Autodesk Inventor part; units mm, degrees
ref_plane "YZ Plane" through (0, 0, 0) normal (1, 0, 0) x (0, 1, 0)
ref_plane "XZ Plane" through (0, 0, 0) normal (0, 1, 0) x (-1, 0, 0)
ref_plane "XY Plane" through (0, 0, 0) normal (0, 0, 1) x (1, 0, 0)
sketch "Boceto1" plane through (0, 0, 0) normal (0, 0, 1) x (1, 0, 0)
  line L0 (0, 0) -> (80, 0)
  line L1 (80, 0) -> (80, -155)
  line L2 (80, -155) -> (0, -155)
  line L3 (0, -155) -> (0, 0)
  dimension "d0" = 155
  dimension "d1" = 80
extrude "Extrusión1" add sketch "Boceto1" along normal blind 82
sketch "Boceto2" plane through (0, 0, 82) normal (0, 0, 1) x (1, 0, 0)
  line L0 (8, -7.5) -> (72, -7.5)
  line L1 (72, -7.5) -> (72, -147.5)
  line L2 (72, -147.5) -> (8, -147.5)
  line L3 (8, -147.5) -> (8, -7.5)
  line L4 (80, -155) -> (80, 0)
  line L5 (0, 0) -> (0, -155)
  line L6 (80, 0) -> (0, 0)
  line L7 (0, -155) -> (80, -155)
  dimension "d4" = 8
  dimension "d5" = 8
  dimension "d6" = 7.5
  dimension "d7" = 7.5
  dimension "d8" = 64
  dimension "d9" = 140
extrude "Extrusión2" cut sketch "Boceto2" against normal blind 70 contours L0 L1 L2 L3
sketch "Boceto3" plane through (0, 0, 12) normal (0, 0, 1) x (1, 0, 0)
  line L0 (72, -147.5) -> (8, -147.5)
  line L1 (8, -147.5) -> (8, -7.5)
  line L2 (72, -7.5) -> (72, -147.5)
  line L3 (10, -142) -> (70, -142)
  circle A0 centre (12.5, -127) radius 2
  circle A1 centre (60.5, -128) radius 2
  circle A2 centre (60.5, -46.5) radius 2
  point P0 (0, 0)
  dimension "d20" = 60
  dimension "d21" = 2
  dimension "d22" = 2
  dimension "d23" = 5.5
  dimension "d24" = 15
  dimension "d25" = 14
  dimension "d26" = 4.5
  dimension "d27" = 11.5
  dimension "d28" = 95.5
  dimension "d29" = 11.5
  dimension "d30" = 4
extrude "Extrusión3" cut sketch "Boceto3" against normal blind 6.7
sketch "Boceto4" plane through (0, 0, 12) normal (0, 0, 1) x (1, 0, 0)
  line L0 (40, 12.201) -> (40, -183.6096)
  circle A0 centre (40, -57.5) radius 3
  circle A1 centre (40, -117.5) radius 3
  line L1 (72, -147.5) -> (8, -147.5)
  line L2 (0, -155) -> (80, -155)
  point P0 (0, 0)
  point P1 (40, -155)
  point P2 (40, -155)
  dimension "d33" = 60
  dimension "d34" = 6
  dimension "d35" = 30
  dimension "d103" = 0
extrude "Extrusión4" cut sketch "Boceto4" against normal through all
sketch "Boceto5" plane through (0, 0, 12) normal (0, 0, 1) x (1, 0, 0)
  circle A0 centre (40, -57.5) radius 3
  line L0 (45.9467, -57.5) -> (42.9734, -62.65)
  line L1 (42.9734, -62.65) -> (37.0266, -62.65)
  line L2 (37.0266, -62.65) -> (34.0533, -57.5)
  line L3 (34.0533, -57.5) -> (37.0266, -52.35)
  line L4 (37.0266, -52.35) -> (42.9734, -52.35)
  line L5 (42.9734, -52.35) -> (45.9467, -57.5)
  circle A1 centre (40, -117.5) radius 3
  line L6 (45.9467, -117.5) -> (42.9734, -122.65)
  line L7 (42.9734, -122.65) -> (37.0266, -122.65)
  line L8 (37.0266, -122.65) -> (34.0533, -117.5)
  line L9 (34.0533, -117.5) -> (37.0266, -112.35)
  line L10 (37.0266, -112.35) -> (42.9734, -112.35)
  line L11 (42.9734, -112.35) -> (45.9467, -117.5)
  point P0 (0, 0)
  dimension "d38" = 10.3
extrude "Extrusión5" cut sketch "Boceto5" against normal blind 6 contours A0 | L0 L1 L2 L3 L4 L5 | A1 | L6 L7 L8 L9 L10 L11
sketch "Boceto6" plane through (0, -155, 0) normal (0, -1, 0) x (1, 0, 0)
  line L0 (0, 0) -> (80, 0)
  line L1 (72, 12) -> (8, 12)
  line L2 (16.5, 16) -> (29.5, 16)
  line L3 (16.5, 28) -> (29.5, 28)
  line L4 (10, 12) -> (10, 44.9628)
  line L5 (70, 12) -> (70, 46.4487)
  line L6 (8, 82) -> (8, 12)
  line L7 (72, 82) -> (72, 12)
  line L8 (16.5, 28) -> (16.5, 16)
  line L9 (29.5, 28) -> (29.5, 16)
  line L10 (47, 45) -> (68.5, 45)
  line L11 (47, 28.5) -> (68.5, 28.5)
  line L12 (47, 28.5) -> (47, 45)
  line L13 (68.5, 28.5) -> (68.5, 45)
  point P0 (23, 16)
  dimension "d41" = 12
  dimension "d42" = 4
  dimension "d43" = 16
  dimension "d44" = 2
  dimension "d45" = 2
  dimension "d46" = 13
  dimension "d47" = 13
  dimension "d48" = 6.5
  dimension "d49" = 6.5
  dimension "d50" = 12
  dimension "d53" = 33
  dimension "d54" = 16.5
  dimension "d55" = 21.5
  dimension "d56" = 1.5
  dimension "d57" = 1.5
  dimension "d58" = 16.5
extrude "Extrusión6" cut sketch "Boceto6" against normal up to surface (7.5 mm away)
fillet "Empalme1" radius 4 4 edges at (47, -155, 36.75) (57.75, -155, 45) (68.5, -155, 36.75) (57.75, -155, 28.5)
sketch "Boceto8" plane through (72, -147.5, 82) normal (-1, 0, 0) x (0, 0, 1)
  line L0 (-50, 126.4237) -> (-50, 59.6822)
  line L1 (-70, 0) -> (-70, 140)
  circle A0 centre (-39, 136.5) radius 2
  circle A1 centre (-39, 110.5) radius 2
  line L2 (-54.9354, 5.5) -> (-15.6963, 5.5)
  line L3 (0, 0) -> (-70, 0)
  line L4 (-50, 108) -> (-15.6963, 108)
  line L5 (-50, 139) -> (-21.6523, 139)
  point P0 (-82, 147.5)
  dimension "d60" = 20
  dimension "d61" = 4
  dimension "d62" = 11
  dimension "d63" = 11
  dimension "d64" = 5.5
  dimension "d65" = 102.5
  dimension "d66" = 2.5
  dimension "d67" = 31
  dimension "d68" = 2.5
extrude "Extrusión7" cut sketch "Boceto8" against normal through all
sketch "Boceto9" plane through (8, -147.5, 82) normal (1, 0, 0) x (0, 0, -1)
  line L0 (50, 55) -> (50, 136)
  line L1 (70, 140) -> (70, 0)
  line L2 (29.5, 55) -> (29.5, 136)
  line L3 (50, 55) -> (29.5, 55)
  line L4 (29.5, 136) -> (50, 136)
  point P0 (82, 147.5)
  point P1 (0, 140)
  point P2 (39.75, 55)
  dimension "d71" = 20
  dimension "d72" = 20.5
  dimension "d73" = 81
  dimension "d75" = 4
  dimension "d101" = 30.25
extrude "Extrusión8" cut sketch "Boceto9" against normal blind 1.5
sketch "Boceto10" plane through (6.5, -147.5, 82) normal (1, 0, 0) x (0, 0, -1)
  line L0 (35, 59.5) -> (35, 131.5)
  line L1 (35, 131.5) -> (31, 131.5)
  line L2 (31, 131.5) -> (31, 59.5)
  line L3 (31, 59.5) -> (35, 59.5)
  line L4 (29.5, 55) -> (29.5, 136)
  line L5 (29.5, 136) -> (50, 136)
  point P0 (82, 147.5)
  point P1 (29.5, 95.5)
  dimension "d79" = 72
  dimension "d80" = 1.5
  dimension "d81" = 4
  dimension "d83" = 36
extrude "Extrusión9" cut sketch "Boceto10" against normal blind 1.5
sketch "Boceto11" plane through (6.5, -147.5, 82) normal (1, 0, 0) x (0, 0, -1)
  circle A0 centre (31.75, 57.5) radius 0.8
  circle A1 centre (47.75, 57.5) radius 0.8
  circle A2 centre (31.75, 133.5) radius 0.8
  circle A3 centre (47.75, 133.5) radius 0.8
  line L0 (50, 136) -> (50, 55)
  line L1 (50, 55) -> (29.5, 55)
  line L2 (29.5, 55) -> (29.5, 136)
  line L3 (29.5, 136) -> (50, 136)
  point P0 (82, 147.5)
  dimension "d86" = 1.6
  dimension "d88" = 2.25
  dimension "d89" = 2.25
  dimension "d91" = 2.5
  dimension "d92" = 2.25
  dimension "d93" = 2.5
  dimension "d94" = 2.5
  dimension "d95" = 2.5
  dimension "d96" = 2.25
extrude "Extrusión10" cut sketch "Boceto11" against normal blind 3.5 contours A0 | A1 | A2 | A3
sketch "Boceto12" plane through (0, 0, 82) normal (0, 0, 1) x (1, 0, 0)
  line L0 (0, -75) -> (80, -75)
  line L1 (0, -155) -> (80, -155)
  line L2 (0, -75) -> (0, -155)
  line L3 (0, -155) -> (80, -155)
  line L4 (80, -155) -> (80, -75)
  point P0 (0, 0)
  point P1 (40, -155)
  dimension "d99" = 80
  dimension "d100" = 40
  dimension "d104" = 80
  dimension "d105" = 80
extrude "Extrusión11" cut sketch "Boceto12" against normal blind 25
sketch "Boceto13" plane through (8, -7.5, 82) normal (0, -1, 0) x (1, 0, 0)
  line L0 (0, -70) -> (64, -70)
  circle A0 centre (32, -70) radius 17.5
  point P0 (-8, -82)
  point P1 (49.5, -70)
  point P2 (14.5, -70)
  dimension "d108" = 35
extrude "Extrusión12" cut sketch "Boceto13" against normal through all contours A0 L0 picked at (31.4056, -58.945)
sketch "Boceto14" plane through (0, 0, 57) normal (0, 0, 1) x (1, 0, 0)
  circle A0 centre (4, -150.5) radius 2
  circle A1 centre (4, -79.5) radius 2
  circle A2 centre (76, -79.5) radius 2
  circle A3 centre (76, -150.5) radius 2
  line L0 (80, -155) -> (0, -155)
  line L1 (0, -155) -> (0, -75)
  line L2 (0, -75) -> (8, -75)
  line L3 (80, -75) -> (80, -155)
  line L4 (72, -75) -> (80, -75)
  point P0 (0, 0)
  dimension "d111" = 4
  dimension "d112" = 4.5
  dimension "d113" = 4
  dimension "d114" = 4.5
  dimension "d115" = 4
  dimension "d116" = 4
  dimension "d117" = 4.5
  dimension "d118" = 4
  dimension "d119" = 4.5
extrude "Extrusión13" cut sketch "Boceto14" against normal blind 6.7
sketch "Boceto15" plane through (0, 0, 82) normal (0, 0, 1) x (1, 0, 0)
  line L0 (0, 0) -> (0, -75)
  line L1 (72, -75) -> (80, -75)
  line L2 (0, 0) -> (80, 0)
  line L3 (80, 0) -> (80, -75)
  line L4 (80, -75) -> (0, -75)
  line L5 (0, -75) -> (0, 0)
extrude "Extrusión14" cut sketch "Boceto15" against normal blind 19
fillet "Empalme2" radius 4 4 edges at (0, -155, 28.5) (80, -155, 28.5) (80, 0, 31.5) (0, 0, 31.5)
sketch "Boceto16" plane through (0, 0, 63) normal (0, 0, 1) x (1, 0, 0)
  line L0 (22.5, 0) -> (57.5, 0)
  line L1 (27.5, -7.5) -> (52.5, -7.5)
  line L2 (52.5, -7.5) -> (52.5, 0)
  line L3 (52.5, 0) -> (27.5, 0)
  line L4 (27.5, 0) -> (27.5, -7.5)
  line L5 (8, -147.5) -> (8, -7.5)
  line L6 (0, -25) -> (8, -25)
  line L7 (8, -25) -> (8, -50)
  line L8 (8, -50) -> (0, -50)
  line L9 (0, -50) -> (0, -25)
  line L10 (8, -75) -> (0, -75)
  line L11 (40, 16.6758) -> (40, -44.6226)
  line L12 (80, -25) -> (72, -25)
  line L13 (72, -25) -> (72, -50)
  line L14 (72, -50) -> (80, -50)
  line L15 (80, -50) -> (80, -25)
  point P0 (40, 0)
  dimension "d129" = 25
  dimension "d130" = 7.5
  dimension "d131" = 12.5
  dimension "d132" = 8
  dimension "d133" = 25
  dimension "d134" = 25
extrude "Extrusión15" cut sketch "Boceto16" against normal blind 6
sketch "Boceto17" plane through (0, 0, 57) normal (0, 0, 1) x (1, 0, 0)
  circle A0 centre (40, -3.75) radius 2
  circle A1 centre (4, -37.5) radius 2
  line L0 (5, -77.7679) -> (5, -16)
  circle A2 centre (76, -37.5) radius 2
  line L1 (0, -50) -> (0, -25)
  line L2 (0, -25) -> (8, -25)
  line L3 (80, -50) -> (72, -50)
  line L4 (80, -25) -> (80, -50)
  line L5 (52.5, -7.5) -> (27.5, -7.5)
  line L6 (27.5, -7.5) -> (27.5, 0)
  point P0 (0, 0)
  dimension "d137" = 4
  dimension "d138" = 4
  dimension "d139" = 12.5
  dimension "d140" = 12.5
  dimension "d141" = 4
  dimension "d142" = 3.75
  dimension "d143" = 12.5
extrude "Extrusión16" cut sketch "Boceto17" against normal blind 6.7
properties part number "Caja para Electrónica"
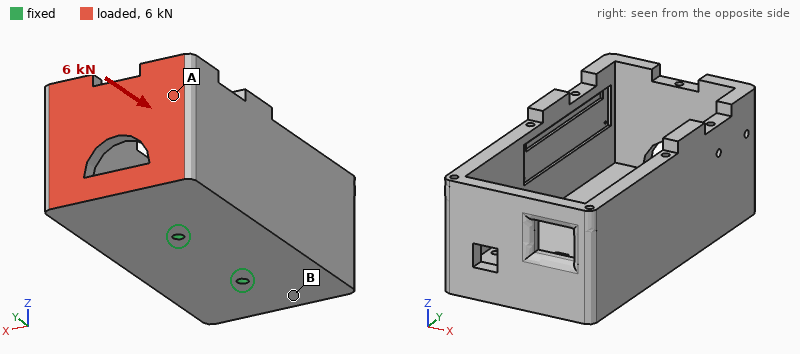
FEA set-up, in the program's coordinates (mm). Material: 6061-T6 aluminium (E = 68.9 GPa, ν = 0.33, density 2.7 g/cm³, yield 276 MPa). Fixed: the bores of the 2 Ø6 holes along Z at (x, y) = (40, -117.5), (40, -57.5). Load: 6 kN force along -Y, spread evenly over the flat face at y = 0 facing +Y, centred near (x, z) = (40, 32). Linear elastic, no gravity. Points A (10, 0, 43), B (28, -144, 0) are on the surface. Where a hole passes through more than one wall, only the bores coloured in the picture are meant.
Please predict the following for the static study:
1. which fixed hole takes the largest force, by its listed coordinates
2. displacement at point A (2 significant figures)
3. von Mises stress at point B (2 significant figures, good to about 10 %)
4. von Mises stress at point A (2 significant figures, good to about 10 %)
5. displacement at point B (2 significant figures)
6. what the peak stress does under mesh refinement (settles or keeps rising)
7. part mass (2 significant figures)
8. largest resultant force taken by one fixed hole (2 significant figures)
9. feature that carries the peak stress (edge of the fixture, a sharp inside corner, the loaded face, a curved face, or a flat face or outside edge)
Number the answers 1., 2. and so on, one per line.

1. (40, -57.5)
2. 0.081 mm
3. 8.9 MPa
4. 19 MPa
5. 0.027 mm
6. keeps rising
7. 800 g
8. 4.2 kN
9. edge of the fixture
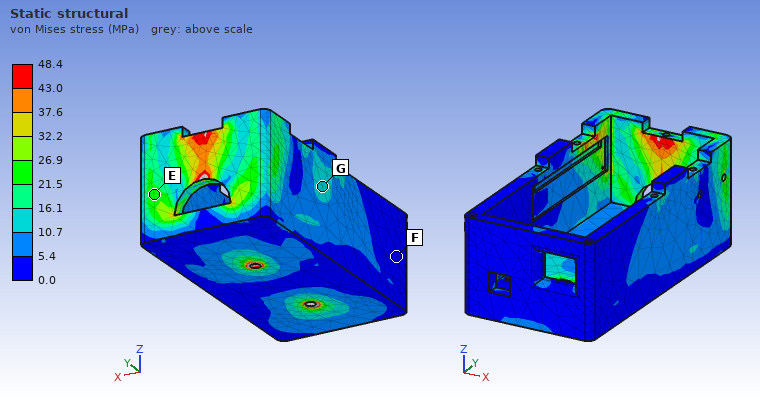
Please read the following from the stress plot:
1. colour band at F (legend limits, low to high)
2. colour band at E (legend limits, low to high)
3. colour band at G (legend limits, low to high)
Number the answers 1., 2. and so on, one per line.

1. 0.0 to 5.4 MPa
2. 21.5 to 26.9 MPa
3. 10.7 to 16.1 MPa
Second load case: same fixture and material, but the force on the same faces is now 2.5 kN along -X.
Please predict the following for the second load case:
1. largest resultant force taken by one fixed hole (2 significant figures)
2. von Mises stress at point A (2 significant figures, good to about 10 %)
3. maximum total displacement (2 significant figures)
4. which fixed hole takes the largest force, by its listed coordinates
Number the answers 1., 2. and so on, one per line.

1. 4.7 kN
2. 12 MPa
3. 0.34 mm
4. (40, -57.5)
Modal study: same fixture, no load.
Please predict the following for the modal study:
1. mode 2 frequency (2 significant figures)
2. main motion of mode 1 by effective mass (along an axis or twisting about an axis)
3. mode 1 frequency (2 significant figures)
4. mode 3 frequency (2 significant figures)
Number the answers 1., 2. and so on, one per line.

1. 1500 Hz
2. along X
3. 720 Hz
4. 1600 Hz
